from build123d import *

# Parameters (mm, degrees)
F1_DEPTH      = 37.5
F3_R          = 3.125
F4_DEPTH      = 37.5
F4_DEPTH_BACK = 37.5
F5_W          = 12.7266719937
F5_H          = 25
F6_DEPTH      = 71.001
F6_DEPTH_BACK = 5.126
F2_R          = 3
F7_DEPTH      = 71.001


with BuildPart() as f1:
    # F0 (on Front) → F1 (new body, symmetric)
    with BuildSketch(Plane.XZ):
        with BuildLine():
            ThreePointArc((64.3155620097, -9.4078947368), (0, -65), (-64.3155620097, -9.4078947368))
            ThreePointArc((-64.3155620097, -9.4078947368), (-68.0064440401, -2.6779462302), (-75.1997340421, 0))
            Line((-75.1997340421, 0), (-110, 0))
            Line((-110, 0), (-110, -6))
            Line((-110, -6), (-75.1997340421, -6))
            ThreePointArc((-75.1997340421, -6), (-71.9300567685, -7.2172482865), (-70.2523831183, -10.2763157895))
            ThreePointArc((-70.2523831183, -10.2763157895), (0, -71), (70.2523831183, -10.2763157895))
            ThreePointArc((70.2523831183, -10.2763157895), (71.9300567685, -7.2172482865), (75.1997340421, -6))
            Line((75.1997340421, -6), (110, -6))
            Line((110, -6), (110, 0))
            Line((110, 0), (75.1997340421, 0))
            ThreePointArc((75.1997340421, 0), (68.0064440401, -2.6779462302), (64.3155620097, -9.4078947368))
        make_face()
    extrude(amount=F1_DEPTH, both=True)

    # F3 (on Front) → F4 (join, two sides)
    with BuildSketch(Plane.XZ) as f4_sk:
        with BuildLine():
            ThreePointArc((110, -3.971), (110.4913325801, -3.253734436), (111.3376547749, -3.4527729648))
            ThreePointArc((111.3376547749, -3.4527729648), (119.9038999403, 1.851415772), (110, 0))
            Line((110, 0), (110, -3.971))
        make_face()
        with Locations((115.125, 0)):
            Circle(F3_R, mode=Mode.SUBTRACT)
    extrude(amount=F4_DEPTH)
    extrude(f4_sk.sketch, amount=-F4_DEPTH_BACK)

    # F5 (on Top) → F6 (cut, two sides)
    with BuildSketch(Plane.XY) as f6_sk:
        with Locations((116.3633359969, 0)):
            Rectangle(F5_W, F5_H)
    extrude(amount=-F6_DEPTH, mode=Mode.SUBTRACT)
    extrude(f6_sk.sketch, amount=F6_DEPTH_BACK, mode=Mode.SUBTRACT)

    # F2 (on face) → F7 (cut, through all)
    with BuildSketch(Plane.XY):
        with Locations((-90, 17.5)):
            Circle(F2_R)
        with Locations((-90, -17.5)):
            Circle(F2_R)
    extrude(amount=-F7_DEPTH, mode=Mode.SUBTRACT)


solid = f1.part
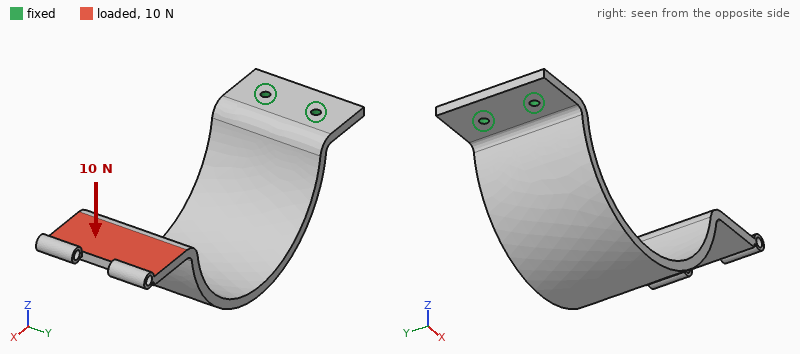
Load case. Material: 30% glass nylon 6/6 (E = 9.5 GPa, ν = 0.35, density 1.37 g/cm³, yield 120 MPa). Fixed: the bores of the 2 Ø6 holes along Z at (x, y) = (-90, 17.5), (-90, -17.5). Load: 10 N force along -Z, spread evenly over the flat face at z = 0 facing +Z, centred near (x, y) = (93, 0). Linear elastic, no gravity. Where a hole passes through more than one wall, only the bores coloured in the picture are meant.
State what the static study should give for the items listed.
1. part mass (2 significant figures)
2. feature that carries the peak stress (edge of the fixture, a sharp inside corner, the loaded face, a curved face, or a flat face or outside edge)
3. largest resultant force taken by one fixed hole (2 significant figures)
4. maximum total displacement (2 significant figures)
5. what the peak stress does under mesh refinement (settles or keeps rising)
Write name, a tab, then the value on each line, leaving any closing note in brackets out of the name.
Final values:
part mass	180 g
feature that carries the peak stress	edge of the fixture
largest resultant force taken by one fixed hole	5.4 N
maximum total displacement	2.6 mm
what the peak stress does under mesh refinement	keeps rising
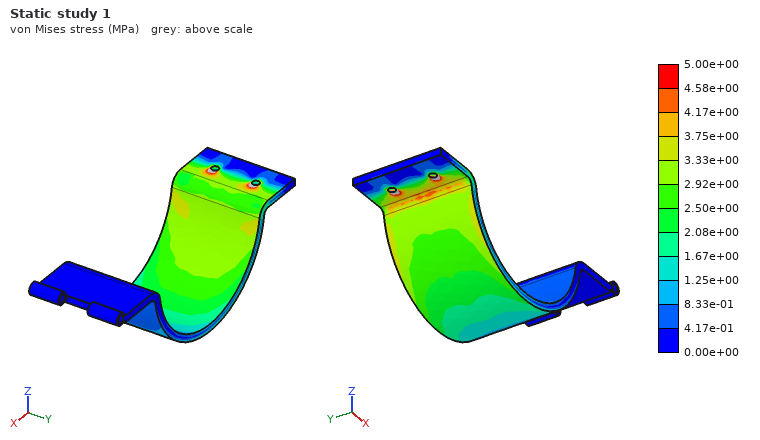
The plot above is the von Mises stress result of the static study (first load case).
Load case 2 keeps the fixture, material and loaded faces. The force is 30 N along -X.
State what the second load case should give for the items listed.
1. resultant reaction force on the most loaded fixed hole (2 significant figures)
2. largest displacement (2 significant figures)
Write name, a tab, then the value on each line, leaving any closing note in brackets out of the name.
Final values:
resultant reaction force on the most loaded fixed hole	15 N
largest displacement	2.7 mm
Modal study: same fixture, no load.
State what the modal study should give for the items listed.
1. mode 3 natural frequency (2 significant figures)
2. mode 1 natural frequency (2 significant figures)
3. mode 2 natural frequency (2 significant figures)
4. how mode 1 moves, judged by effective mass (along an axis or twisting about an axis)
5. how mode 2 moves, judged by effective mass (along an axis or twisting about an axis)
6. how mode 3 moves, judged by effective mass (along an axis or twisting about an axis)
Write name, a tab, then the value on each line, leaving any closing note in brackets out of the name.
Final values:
mode 3 natural frequency	140 Hz
mode 1 natural frequency	45 Hz
mode 2 natural frequency	78 Hz
how mode 1 moves, judged by effective mass	along Z
how mode 2 moves, judged by effective mass	along Y
how mode 3 moves, judged by effective mass	along X
